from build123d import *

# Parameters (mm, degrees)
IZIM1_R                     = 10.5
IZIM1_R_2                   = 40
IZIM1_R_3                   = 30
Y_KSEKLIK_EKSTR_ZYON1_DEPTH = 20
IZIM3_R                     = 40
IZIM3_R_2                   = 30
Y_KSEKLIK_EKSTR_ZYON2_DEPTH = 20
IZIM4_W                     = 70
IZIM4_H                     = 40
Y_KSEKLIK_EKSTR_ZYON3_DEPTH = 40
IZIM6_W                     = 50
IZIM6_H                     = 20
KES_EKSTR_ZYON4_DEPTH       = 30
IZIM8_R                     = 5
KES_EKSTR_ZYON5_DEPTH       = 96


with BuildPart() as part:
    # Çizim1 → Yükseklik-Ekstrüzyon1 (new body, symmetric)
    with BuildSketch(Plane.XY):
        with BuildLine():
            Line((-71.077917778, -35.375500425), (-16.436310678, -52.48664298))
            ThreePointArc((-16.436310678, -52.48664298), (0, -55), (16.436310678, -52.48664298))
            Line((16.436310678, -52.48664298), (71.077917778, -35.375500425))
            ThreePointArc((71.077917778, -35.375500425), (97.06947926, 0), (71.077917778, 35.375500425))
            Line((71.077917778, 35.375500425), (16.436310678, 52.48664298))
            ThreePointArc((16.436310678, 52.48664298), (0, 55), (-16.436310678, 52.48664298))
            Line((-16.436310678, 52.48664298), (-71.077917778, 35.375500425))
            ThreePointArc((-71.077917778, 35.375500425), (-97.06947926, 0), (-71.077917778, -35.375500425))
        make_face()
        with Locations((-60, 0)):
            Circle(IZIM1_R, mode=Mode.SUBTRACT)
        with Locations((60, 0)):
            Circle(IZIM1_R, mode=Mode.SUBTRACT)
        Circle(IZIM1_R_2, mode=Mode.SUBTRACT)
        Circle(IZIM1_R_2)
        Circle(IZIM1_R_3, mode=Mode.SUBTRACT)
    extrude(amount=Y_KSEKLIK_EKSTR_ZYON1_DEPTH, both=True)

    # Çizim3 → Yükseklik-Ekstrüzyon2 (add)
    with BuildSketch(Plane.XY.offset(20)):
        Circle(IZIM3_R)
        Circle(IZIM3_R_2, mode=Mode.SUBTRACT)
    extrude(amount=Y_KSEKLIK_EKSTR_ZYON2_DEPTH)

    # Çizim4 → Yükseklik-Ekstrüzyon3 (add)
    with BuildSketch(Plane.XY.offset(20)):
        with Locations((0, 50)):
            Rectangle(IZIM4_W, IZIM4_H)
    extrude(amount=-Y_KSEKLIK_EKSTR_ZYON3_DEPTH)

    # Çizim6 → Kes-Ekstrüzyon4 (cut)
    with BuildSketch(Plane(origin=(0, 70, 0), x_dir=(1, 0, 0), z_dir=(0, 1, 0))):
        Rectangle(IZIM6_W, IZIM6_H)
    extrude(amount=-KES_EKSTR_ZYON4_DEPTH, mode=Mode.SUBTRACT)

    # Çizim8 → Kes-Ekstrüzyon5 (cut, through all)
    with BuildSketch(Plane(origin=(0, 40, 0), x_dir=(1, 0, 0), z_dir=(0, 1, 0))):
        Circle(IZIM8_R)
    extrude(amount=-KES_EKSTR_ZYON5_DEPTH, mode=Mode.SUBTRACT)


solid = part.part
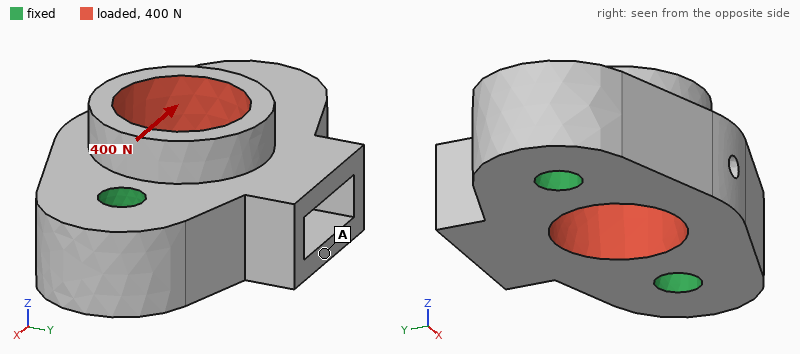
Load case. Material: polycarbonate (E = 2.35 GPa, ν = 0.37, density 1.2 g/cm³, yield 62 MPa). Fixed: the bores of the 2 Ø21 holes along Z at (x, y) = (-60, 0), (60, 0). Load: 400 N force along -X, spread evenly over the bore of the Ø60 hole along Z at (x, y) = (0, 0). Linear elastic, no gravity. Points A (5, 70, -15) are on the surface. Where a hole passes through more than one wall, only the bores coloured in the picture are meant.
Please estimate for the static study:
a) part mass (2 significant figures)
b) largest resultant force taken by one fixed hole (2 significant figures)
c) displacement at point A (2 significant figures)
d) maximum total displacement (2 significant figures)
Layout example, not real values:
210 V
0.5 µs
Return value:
670 g
200 N
0.84 µm
4.8 µm
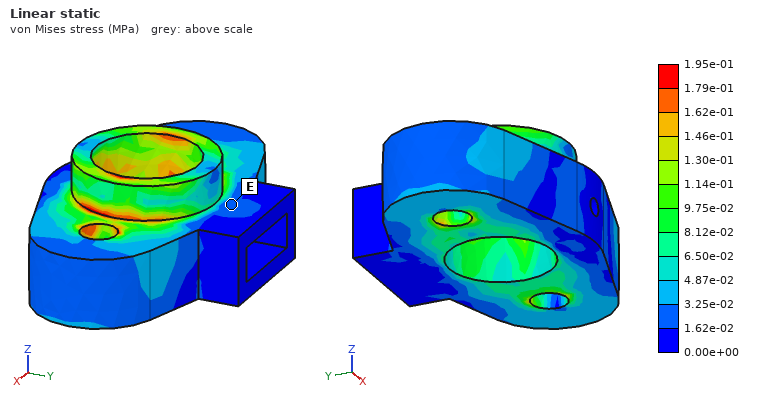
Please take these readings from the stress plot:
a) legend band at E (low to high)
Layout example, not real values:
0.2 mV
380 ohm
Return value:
1.62e-02 to 3.25e-02 MPa
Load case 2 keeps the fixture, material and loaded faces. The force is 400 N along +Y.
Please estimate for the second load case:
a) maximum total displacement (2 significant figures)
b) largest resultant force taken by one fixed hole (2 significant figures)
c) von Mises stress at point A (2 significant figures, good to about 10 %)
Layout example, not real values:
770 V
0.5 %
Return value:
9.2 µm
200 N
0.060 MPa
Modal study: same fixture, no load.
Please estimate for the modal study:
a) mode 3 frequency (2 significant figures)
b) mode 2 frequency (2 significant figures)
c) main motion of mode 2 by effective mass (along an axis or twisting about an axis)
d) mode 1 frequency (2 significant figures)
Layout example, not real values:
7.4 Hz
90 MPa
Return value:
2600 Hz
2000 Hz
along Z
1600 Hz
